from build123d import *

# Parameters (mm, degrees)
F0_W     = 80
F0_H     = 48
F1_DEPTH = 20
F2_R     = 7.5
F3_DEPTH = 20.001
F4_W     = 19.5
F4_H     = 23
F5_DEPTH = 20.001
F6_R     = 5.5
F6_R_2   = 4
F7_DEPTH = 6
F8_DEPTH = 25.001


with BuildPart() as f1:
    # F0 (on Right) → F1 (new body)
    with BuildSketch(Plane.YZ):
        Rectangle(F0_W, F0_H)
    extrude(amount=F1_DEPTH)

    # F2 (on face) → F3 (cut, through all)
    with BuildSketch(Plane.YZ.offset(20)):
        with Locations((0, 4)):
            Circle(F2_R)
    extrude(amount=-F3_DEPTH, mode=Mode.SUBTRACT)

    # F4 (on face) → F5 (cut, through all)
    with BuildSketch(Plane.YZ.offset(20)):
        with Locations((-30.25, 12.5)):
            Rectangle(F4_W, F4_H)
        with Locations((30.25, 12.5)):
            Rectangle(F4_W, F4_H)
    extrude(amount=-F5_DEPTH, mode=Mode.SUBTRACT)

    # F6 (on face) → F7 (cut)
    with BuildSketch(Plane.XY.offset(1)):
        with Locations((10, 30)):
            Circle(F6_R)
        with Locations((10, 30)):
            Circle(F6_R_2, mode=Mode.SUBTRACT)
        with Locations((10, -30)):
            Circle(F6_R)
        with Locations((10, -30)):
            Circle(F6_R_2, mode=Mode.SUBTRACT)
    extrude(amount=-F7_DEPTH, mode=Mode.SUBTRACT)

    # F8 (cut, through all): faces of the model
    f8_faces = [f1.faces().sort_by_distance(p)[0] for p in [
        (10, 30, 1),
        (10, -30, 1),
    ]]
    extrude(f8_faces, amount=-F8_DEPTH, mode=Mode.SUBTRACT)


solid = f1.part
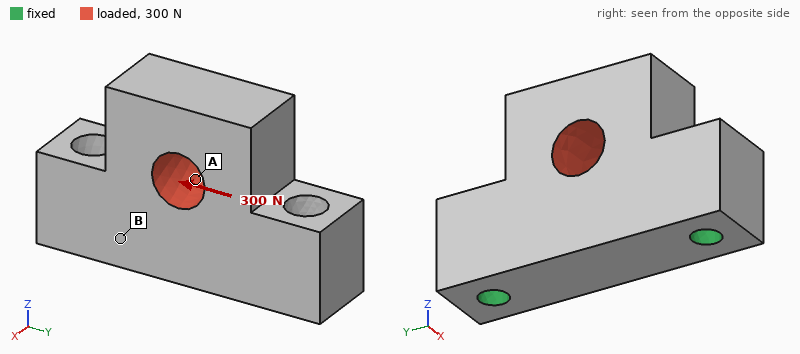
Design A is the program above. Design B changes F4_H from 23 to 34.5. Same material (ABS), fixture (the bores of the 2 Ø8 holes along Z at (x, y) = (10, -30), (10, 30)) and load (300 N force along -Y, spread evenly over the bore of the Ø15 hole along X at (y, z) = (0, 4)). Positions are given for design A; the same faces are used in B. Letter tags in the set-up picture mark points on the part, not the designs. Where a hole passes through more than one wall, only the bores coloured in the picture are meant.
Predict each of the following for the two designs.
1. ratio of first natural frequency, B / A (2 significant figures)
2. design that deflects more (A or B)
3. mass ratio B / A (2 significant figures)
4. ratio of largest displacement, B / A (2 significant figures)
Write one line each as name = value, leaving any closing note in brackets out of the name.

ratio of first natural frequency, B / A = 0.86
design that deflects more = B
mass ratio B / A = 0.94
ratio of largest displacement, B / A = 1.6
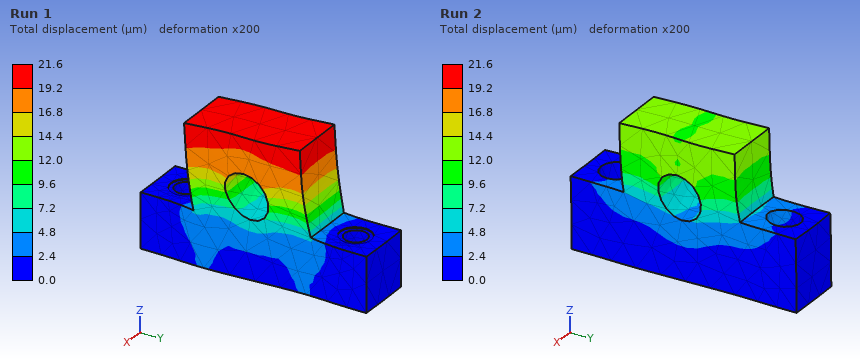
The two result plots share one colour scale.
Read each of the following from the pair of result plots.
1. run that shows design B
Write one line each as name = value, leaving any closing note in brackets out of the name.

run that shows design B = Run 1
